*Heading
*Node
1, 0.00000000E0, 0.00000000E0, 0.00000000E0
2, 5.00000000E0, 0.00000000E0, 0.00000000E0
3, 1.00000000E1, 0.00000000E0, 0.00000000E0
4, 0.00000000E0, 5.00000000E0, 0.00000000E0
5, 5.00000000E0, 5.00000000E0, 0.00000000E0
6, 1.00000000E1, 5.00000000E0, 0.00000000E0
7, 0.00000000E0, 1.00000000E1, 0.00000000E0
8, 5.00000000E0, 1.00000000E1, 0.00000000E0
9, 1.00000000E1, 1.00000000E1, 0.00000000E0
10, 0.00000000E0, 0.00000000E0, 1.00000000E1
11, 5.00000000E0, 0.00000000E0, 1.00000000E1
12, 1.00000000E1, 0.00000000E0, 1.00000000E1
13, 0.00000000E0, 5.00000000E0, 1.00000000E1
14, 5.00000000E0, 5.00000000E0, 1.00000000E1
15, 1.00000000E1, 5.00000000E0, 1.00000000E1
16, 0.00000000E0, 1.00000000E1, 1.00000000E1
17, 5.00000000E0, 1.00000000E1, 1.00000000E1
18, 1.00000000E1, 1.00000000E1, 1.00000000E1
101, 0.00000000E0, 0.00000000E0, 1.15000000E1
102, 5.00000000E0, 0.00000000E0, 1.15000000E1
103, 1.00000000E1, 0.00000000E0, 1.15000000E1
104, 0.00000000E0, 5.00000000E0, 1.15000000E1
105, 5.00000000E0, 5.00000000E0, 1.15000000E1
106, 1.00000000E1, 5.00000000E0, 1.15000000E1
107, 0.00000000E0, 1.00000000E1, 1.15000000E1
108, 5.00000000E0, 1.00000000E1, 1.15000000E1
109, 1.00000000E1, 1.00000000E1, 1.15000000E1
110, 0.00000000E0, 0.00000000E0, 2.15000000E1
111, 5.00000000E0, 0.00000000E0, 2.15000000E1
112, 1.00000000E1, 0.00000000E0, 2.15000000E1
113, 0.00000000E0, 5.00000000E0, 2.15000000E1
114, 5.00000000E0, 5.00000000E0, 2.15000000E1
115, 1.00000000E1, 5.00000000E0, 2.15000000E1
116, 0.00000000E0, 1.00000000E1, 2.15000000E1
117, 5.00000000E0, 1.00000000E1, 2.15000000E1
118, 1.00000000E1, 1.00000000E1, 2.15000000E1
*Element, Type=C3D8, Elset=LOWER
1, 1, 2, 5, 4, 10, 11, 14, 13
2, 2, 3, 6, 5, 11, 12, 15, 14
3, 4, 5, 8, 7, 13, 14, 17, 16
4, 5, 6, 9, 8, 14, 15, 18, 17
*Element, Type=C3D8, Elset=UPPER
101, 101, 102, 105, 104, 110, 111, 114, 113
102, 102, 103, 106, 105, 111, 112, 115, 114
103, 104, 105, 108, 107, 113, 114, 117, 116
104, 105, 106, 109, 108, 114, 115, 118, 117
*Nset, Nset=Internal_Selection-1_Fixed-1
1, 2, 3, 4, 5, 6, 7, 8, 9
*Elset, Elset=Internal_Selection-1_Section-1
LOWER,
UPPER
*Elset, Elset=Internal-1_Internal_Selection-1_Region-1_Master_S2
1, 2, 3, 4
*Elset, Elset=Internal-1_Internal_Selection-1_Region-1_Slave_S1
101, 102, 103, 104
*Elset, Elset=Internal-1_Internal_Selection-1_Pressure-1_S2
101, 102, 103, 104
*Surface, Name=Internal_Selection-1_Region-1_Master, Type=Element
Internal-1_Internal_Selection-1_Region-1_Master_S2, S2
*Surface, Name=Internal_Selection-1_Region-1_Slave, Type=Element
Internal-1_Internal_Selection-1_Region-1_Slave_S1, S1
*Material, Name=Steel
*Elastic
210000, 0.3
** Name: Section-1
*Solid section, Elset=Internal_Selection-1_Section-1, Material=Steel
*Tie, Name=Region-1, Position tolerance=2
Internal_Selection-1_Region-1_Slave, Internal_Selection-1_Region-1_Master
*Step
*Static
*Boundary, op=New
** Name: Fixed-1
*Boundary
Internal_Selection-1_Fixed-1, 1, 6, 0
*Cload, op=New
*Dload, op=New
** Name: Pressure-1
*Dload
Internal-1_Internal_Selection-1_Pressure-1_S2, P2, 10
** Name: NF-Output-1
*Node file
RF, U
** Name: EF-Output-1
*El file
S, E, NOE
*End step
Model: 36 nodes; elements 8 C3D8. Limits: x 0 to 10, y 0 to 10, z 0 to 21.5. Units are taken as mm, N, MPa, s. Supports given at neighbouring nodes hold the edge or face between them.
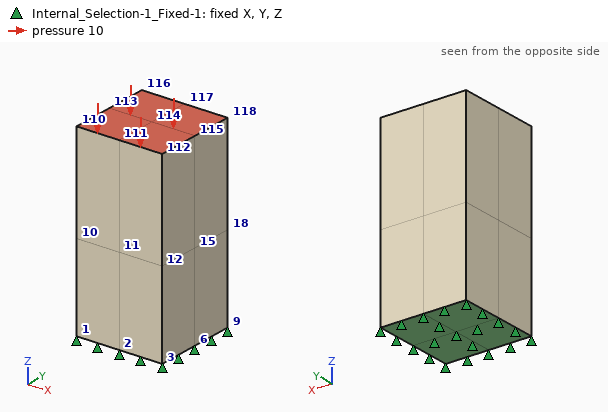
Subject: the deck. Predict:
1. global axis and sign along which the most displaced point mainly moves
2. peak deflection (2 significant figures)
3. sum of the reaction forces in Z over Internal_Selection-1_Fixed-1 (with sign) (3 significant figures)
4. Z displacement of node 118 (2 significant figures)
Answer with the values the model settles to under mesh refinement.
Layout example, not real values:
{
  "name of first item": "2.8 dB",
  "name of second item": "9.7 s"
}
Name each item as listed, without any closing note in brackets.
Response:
{
  "global axis and sign along which the most displaced point mainly moves": "-Z",
  "peak deflection": "0.0010 mm",
  "sum of the reaction forces in Z over Internal_Selection-1_Fixed-1 (with sign)": "1000 N",
  "Z displacement of node 118": "-1.0e-03 mm"
}
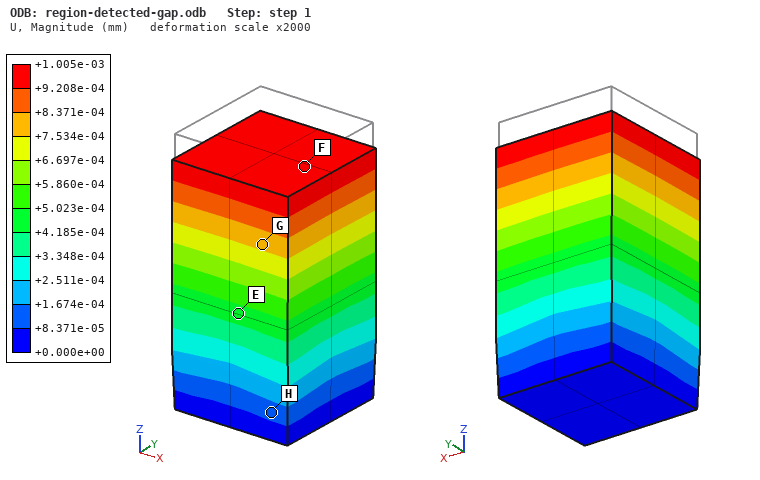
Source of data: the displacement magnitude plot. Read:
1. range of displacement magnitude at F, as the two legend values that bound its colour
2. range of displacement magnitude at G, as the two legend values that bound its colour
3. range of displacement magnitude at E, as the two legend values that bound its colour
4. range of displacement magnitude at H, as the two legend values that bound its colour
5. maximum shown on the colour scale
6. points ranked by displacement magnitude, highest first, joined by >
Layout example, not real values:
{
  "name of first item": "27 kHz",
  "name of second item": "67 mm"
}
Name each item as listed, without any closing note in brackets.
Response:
{
  "range of displacement magnitude at F, as the two legend values that bound its colour": "+9.208e-04 to +1.005e-03 mm",
  "range of displacement magnitude at G, as the two legend values that bound its colour": "+7.534e-04 to +8.371e-04 mm",
  "range of displacement magnitude at E, as the two legend values that bound its colour": "+4.185e-04 to +5.023e-04 mm",
  "range of displacement magnitude at H, as the two legend values that bound its colour": "+8.371e-05 to +1.674e-04 mm",
  "maximum shown on the colour scale": "+1.005e-03 mm",
  "points ranked by displacement magnitude, highest first, joined by >": "F > G > E > H"
}
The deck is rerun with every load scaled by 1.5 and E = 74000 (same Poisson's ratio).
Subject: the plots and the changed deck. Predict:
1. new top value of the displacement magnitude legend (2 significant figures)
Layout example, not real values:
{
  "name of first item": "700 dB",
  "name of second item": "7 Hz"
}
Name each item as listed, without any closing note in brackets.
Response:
{
  "new top value of the displacement magnitude legend": "0.0043 mm"
}
